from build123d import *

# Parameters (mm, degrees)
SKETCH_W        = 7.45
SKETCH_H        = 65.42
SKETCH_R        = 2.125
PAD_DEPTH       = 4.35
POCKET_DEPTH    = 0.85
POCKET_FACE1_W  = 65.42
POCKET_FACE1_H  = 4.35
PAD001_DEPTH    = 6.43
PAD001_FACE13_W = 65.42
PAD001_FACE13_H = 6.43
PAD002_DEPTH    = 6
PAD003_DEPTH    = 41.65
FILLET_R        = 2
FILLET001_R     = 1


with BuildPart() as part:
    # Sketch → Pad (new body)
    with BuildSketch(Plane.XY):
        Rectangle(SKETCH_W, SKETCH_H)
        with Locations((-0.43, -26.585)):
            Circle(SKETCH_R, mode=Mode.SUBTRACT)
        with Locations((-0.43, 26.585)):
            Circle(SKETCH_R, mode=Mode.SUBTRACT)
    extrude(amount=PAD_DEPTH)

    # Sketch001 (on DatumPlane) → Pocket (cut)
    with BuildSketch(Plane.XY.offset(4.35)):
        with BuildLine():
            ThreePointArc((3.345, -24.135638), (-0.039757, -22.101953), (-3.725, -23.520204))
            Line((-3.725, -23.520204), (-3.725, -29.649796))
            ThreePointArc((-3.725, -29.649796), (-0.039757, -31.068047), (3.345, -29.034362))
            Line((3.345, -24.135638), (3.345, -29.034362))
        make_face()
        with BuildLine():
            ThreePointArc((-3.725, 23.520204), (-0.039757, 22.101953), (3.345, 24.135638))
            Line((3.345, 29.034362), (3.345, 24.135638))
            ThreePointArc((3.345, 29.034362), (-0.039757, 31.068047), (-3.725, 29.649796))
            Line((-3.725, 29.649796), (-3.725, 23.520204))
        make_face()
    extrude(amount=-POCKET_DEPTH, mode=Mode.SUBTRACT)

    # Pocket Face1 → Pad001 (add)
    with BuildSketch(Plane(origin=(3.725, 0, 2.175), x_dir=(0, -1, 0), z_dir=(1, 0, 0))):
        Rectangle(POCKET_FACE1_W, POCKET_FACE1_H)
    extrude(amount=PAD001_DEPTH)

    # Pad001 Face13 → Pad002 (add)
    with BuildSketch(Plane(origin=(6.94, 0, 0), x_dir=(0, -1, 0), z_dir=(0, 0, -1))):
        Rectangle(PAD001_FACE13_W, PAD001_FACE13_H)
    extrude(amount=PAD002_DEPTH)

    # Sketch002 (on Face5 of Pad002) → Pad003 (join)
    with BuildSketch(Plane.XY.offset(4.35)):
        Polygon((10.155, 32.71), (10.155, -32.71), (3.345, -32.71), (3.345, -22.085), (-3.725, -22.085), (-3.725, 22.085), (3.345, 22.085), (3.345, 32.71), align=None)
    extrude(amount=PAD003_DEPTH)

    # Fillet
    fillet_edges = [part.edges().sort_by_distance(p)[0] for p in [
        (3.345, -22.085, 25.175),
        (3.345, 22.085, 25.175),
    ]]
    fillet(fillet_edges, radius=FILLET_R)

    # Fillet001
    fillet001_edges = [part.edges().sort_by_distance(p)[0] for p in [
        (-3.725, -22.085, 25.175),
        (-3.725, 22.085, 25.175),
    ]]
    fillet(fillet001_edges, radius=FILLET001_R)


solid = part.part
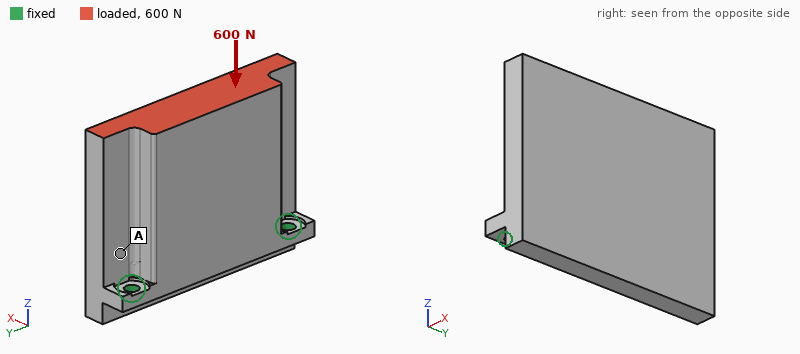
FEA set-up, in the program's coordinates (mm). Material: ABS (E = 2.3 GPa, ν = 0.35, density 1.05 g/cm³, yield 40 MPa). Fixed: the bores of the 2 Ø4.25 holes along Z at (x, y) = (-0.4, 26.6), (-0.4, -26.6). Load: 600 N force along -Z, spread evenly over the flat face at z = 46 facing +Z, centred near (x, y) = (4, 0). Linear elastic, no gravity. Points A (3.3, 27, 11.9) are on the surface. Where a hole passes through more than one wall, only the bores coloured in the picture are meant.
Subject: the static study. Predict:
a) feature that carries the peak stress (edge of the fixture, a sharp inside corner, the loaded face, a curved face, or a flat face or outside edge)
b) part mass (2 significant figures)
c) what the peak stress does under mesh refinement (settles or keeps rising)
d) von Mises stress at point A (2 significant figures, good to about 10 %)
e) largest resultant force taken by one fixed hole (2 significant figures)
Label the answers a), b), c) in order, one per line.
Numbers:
a) edge of the fixture
b) 40 g
c) keeps rising
d) 3.4 MPa
e) 300 N
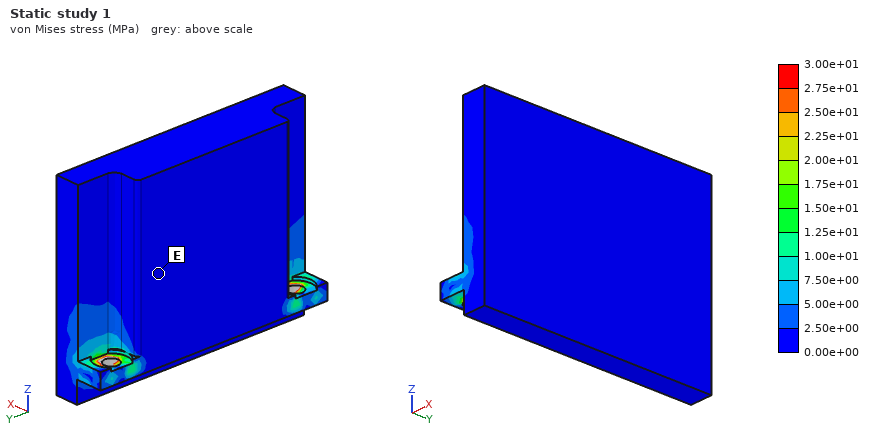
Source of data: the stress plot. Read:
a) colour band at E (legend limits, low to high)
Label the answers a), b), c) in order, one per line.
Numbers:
a) 0.00e+00 to 2.50e+00 MPa
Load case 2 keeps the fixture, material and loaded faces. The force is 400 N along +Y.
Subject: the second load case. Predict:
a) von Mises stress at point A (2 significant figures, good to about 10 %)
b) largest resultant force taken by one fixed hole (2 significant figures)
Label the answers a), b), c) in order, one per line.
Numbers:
a) 3.9 MPa
b) 400 N
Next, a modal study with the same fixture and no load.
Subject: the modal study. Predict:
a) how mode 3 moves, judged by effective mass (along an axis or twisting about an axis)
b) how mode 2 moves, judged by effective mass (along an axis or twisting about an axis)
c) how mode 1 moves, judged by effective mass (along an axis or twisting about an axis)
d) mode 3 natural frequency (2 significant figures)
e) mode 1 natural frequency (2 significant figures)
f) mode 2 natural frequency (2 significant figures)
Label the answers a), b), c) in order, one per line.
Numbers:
a) along Y
b) along Y
c) along X
d) 2200 Hz
e) 320 Hz
f) 1900 Hz
